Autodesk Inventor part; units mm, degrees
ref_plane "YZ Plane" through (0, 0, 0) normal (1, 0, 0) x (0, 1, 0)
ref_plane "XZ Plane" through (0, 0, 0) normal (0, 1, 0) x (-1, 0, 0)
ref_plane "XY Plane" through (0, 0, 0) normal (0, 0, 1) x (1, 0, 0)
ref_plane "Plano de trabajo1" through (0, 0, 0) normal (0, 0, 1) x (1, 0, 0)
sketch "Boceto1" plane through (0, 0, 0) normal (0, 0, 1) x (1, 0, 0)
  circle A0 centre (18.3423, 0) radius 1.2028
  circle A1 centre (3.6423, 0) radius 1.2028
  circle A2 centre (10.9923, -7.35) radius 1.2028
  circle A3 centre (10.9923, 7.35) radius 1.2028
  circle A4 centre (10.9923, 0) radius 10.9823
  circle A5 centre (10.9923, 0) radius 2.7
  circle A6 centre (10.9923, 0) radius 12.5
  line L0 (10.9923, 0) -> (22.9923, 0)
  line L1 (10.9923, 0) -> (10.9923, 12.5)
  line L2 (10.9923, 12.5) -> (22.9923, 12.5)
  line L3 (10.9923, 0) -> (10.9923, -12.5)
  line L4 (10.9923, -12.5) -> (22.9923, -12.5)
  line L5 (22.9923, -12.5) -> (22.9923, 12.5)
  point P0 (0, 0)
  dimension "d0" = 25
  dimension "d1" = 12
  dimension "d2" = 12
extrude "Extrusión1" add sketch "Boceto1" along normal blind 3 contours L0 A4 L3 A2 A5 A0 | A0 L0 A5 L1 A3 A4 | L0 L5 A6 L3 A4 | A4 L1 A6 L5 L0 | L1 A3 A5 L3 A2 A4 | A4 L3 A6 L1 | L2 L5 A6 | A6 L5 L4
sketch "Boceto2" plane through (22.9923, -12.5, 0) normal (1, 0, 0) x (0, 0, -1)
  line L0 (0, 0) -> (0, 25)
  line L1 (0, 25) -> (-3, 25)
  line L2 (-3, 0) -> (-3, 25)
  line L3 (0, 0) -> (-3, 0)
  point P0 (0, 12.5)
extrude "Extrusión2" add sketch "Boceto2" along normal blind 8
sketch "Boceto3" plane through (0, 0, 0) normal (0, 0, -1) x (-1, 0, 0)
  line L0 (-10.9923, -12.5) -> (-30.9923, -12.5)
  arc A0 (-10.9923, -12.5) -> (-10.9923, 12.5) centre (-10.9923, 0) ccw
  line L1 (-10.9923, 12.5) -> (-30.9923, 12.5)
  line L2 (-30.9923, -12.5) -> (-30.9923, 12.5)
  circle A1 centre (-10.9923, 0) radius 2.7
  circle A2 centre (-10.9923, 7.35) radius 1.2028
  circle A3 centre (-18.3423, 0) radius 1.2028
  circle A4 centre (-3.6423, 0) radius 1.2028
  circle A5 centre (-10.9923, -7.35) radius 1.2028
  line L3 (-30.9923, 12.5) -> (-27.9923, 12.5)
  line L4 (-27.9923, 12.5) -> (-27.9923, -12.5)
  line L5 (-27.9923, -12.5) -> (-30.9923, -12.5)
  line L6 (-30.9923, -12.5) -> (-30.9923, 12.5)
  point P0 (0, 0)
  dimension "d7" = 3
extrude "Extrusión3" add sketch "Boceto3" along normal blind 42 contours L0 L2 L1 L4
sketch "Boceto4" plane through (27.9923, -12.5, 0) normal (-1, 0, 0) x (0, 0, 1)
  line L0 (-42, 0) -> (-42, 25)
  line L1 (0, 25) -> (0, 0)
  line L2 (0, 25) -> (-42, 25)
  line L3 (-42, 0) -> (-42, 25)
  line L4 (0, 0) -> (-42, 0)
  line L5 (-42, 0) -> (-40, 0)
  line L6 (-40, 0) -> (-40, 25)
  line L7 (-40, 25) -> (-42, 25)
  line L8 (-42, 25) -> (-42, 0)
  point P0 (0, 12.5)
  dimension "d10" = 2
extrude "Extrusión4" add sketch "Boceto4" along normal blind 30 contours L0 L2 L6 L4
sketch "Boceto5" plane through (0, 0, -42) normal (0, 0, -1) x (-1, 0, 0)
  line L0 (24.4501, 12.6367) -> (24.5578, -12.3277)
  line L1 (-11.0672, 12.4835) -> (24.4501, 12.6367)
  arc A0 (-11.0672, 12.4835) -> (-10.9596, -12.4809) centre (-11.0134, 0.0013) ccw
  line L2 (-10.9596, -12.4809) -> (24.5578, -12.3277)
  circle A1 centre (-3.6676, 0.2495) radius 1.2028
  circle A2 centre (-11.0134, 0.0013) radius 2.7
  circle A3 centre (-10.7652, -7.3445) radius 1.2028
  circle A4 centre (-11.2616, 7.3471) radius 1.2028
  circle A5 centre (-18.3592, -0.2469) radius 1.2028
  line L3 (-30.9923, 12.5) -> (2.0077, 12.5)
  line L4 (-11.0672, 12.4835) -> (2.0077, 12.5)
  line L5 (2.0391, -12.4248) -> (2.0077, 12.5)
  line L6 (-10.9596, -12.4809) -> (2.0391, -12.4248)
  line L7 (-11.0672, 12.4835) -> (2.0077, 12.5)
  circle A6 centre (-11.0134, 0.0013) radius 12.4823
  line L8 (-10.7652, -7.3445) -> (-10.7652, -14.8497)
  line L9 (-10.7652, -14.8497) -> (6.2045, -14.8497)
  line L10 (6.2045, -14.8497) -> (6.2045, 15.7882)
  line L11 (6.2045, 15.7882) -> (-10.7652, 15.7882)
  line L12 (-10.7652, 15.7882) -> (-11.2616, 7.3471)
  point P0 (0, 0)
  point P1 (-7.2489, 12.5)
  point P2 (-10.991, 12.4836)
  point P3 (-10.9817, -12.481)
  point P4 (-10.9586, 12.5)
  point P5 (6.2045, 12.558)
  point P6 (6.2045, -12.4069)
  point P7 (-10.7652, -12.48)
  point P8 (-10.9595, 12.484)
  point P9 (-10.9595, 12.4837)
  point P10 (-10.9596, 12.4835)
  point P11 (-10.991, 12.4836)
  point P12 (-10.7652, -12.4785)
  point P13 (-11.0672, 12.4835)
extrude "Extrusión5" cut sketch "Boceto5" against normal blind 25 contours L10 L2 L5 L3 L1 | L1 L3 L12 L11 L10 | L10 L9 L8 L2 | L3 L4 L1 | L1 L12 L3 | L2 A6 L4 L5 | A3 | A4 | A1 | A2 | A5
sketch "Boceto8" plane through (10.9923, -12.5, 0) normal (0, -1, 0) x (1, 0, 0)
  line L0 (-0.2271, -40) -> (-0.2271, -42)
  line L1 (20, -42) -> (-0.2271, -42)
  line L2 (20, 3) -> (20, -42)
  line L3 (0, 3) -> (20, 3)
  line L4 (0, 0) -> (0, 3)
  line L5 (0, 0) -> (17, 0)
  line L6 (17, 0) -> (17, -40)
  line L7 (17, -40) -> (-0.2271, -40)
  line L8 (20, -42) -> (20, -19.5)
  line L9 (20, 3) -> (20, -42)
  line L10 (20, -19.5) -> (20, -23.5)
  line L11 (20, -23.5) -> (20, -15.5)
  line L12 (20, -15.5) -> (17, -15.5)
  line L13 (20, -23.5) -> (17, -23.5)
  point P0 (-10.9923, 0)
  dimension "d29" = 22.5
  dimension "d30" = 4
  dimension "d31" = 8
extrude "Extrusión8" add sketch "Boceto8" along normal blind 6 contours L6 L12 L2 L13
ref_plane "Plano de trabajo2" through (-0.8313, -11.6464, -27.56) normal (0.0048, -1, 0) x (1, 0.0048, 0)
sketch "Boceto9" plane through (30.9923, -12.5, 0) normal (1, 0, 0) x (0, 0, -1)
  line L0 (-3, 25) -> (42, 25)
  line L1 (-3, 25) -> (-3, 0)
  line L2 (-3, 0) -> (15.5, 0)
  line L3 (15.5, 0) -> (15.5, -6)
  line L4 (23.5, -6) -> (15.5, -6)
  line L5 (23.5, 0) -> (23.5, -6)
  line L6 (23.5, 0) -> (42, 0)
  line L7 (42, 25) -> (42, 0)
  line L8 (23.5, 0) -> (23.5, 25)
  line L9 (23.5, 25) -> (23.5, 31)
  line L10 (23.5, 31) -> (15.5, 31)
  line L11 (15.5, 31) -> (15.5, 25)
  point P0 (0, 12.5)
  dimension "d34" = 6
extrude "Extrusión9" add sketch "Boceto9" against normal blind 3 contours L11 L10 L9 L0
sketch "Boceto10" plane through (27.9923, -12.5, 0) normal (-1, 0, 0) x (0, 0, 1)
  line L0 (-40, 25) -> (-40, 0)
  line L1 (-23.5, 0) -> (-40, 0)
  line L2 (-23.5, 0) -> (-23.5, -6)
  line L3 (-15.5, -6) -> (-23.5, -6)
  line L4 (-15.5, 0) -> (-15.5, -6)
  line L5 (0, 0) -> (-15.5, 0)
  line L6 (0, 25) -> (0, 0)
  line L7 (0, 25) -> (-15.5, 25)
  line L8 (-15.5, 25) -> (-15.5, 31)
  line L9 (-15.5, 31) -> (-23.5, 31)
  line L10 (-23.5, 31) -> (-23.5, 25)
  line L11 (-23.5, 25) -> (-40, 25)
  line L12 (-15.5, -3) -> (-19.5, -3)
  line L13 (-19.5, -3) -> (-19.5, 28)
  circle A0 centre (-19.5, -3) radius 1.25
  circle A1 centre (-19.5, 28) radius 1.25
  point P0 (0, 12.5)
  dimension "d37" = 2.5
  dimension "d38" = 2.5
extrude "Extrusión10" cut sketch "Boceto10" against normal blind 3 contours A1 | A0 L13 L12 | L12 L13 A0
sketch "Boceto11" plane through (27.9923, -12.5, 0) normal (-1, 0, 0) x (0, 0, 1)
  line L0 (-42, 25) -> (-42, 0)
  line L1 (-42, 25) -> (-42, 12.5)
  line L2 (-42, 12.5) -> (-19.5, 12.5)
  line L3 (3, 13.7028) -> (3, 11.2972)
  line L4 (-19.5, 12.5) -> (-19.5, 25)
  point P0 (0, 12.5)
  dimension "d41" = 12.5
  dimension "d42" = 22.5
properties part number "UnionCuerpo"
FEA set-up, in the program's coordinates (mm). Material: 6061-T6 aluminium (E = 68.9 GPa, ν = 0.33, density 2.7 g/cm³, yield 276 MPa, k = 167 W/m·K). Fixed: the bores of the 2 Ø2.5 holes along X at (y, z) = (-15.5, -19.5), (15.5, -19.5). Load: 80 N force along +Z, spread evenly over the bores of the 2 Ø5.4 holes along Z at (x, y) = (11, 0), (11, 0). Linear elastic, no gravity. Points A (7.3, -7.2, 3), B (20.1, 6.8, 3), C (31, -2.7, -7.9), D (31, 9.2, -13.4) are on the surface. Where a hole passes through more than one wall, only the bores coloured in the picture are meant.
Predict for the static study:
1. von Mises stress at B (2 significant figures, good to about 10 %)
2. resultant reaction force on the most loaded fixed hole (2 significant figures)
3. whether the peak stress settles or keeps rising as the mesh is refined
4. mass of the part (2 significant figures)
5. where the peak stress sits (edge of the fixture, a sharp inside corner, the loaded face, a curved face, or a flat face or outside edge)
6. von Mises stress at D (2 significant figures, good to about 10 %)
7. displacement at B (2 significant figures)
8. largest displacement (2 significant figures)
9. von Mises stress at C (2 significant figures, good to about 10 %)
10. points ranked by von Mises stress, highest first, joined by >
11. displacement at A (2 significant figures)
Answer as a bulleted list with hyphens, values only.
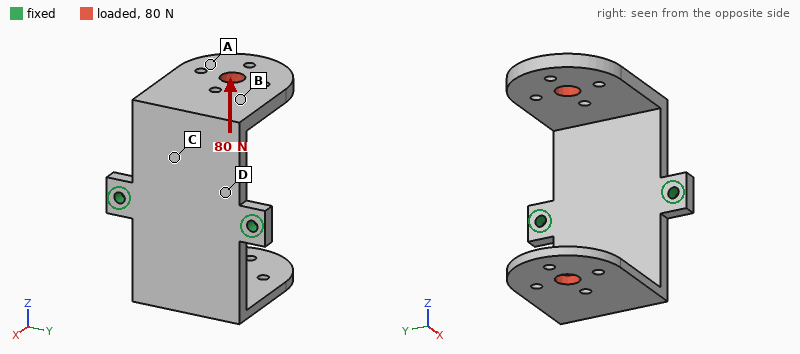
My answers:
- 11 MPa
- 40 N
- keeps rising
- 18 g
- edge of the fixture
- 27 MPa
- 0.12 mm
- 0.28 mm
- 21 MPa
- D > C > B > A
- 0.20 mm
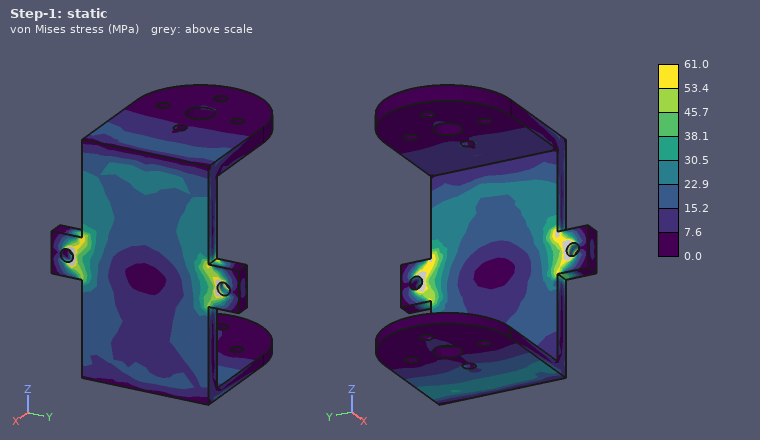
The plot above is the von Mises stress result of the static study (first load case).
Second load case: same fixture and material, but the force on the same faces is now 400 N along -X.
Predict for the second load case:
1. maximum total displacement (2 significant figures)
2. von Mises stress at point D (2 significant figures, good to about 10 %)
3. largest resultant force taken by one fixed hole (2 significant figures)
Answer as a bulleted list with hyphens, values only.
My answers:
- 0.53 mm
- 100 MPa
- 200 N
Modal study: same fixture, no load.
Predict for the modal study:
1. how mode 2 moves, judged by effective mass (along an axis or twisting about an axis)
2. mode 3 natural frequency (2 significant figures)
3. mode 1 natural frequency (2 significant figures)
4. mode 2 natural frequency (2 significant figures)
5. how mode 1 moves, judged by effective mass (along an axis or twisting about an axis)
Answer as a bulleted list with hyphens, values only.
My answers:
- along X
- 2400 Hz
- 1100 Hz
- 1400 Hz
- along Z
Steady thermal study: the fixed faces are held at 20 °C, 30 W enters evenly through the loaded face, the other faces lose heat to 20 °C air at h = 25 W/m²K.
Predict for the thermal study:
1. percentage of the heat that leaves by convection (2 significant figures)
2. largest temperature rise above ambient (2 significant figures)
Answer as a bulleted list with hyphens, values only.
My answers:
- 18 %
- 70 K
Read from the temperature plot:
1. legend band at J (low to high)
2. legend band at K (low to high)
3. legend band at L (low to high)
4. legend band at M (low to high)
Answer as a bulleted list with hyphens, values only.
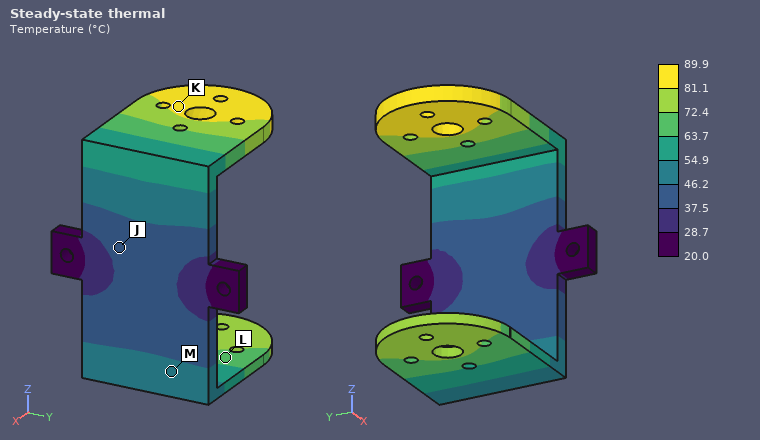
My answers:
- 37.5 to 46.2 °C
- 81.1 to 89.9 °C
- 63.7 to 72.4 °C
- 46.2 to 54.9 °C
